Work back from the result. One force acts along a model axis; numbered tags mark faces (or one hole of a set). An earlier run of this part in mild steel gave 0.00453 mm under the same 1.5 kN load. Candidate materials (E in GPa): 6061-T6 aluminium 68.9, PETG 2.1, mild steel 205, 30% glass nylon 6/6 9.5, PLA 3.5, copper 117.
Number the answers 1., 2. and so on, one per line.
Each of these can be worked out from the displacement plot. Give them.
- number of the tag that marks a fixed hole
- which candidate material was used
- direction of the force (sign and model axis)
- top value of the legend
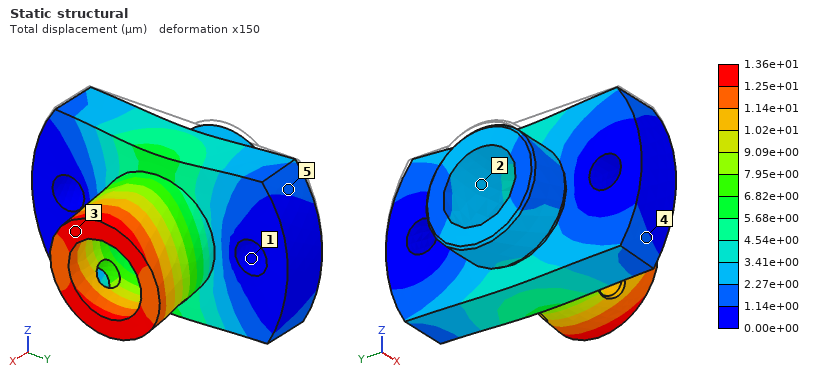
1. 1
2. 6061-T6 aluminium
3. -Z
4. 1.36e+01 µm
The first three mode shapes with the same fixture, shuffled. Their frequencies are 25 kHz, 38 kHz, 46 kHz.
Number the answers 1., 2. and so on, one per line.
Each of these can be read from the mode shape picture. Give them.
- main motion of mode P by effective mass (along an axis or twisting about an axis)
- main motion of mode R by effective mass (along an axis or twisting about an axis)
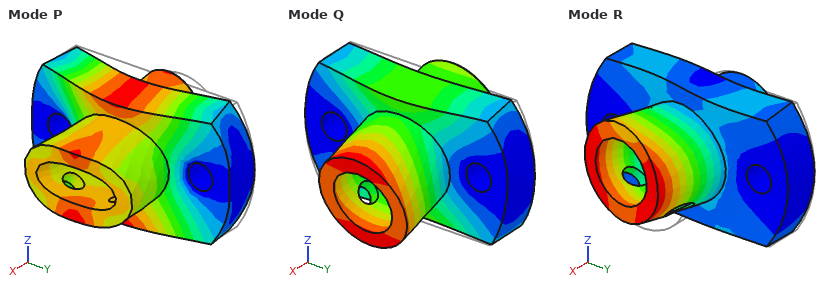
1. along X
2. along Y
